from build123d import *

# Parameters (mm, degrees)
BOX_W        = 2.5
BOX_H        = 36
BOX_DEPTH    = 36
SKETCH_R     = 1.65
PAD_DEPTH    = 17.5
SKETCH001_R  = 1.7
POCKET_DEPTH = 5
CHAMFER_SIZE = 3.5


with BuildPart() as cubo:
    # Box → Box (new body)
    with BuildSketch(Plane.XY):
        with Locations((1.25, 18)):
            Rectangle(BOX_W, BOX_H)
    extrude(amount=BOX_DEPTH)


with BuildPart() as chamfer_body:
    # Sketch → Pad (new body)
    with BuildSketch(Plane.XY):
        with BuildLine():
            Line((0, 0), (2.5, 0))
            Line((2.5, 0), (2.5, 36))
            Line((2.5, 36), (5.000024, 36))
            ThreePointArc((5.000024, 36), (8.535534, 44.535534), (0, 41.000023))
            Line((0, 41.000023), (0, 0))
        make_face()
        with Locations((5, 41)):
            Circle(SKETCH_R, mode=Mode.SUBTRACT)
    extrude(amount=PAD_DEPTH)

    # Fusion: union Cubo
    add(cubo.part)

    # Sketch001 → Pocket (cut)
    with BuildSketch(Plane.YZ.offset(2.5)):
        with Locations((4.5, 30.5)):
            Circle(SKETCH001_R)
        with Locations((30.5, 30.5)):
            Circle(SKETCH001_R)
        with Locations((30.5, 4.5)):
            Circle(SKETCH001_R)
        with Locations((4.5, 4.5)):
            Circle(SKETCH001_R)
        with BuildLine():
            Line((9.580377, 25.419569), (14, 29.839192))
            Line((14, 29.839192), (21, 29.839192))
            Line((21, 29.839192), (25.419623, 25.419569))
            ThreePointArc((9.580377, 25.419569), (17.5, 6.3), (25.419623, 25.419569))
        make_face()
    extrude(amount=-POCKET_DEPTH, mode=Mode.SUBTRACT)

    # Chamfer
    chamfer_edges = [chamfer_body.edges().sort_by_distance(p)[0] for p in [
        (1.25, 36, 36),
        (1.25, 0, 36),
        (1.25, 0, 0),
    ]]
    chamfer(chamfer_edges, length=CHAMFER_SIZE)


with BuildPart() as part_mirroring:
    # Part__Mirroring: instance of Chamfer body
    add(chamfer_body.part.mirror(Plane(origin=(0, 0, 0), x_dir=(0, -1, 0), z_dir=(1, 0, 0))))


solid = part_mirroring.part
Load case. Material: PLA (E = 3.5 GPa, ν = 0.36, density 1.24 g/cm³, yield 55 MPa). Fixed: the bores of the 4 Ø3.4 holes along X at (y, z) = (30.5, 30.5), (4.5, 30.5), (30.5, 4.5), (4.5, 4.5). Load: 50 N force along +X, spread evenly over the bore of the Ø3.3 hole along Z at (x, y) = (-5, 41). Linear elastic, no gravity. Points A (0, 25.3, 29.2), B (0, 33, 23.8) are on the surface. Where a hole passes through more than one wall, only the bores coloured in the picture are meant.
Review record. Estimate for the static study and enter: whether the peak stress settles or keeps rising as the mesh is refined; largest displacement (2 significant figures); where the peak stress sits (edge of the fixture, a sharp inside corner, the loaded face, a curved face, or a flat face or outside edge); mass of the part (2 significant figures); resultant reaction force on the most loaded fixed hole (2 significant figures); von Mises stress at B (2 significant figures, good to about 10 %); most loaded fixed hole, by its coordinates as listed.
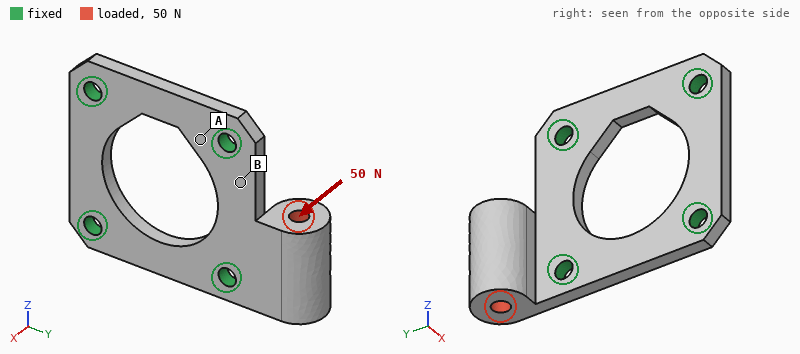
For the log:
keeps rising
0.44 mm
edge of the fixture
4.2 g
44 N
8.1 MPa
(30.5, 4.5)
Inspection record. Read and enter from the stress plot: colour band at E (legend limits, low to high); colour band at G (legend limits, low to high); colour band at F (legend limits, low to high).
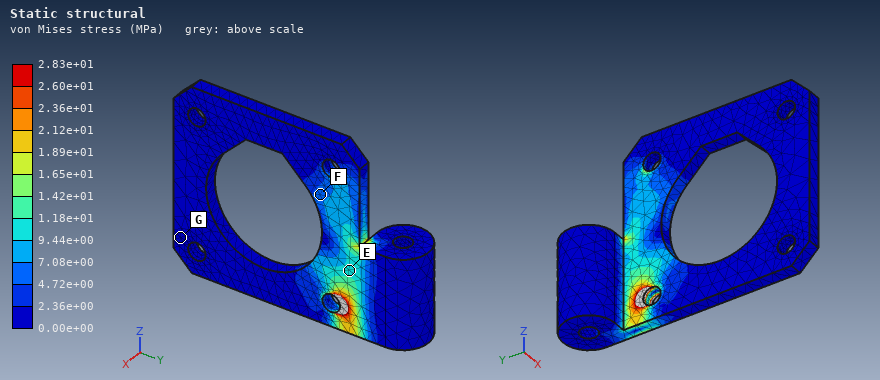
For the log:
9.44e+00 to 1.18e+01 MPa
0.00e+00 to 2.36e+00 MPa
4.72e+00 to 7.08e+00 MPa
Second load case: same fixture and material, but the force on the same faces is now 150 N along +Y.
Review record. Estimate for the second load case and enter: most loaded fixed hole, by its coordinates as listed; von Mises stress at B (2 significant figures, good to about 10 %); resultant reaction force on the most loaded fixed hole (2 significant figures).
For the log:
(30.5, 4.5)
7.8 MPa
130 N
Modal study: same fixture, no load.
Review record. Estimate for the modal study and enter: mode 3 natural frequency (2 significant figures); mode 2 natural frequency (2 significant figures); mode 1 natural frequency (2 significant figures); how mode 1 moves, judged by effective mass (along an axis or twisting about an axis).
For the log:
6400 Hz
3600 Hz
1500 Hz
along X
